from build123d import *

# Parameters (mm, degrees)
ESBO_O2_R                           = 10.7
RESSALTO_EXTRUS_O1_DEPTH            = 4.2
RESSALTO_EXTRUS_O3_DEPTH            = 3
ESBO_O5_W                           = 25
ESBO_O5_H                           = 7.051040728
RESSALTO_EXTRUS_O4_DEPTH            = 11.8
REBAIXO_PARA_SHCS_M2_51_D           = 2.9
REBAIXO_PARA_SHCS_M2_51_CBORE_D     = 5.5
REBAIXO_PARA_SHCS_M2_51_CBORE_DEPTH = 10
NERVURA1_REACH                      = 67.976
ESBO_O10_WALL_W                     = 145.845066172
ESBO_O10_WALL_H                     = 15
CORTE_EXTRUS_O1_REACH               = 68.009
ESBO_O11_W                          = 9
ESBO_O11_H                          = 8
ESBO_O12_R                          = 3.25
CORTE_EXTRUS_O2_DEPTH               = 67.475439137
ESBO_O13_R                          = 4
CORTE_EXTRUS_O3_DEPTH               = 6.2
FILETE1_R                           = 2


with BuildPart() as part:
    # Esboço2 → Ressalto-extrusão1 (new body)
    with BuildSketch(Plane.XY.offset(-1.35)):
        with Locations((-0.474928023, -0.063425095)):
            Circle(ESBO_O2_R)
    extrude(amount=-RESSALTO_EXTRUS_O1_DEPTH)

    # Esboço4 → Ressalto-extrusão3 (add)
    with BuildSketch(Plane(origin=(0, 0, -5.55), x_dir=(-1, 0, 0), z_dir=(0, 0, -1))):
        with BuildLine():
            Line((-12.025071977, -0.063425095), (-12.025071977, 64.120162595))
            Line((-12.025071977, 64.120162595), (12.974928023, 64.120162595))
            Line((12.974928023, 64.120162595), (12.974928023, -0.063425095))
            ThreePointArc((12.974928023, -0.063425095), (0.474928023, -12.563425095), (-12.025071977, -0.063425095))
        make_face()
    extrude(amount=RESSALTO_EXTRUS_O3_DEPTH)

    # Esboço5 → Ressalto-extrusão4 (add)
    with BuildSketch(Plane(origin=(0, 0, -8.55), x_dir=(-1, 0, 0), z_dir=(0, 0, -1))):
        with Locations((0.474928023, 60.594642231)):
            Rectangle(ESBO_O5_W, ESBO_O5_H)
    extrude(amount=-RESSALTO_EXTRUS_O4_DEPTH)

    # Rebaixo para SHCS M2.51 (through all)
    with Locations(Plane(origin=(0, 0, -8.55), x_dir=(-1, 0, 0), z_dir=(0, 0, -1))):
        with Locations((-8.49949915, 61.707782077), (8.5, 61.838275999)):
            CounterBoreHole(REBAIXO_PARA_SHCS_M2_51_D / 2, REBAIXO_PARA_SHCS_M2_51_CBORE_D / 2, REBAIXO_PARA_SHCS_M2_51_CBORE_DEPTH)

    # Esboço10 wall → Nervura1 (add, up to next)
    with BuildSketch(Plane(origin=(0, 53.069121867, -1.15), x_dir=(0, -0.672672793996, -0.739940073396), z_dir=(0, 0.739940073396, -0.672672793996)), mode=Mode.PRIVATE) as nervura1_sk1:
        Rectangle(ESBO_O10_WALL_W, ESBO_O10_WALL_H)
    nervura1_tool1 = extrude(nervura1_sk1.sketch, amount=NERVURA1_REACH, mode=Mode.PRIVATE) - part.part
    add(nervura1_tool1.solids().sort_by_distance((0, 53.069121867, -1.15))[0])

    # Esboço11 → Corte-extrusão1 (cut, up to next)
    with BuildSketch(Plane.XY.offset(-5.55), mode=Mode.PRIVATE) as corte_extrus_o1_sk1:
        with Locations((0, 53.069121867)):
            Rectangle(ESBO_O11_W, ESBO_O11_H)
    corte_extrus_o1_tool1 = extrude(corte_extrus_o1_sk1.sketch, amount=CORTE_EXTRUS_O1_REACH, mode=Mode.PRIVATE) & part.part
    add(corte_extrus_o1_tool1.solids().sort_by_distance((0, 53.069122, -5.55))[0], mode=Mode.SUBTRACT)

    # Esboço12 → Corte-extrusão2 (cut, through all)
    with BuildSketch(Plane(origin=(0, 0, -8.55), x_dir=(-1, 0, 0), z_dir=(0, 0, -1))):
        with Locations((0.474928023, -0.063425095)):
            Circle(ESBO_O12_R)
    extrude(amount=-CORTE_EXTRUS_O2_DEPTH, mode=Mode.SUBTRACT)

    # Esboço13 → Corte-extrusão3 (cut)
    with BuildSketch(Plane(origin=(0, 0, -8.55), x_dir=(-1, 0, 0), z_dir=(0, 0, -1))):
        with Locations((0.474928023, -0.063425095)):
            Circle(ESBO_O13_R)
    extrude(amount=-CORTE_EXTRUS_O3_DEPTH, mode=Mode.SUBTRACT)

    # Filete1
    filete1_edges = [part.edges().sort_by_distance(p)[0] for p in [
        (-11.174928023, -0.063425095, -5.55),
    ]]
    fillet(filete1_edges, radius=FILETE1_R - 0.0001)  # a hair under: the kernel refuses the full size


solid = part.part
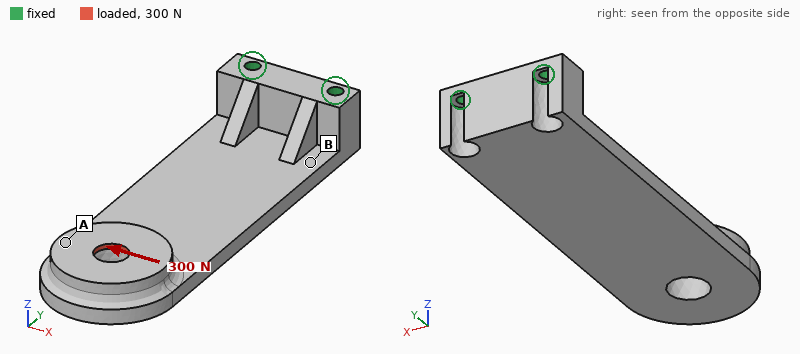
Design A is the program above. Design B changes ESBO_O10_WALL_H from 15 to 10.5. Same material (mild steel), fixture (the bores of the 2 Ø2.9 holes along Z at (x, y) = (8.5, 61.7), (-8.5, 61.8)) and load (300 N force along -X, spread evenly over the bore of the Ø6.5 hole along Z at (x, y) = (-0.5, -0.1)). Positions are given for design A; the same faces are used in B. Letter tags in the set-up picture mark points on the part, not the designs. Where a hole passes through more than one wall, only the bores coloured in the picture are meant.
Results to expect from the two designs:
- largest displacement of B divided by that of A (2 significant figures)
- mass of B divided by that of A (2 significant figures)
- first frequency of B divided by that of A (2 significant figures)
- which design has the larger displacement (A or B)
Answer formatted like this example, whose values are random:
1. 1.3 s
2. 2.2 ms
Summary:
1. 1.2
2. 0.98
3. 0.95
4. B
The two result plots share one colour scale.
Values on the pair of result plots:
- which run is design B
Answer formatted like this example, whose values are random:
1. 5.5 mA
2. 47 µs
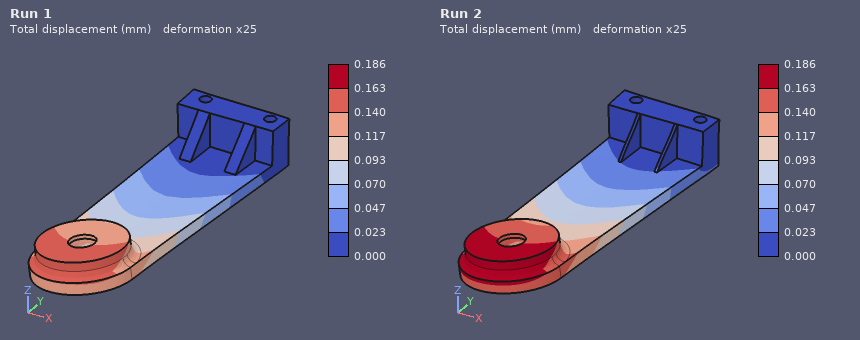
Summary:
1. Run 2
